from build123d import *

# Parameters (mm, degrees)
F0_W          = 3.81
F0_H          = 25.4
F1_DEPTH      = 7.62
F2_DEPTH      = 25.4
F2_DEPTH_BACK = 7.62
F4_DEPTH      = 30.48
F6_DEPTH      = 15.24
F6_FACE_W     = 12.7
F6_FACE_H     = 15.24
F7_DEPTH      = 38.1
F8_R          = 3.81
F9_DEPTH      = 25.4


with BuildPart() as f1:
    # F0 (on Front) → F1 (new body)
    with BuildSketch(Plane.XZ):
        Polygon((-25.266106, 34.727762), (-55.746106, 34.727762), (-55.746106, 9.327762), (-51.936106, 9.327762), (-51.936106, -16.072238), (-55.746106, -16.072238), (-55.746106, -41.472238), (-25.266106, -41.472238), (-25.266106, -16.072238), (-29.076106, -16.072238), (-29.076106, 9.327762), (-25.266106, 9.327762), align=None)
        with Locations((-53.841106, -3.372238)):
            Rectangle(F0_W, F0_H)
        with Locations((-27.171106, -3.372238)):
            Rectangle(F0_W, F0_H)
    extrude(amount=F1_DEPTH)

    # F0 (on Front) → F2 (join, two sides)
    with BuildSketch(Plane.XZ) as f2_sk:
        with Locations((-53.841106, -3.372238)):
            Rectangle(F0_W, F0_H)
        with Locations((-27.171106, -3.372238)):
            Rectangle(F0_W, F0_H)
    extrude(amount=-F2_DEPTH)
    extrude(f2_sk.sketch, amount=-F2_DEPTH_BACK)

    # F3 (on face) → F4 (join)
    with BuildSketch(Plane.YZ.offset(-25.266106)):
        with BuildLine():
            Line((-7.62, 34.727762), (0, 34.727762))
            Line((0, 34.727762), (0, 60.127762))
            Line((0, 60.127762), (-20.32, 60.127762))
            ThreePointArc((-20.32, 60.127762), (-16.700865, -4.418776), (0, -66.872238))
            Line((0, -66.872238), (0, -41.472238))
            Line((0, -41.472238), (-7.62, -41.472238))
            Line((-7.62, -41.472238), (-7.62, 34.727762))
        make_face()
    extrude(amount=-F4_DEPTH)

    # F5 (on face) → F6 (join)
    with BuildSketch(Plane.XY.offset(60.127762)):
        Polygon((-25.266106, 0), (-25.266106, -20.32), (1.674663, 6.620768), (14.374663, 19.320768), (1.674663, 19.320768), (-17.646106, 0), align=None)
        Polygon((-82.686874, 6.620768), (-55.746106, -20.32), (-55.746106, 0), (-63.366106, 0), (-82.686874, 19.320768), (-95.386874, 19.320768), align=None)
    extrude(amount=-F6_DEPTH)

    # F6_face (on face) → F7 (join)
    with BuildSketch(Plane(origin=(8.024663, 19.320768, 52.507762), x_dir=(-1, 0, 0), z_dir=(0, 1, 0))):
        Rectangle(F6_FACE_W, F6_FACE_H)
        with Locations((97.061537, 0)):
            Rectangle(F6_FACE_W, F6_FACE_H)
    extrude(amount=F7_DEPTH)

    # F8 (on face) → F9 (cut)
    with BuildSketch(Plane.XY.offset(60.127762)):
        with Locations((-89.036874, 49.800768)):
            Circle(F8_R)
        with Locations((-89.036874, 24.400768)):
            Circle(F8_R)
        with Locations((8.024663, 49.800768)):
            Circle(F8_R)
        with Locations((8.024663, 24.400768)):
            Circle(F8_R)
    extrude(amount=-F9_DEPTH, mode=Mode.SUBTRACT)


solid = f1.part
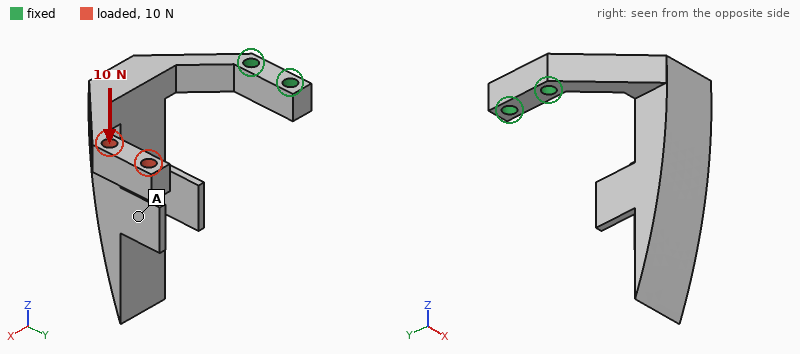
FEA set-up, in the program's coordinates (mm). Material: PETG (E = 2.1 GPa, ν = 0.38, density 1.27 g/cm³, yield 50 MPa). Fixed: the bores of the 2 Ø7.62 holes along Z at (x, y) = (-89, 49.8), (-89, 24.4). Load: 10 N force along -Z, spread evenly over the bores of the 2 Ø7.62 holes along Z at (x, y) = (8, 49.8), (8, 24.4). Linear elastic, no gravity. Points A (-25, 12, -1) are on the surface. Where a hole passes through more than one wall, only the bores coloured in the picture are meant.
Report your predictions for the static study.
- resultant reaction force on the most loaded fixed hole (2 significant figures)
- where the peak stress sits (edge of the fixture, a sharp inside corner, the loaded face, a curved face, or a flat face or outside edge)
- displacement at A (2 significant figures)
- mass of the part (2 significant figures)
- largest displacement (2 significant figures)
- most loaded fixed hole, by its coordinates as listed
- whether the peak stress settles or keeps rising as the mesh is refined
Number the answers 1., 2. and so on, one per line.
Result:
1. 9.7 N
2. edge of the fixture
3. 1.2 mm
4. 110 g
5. 2.1 mm
6. (-89, 24.4)
7. keeps rising
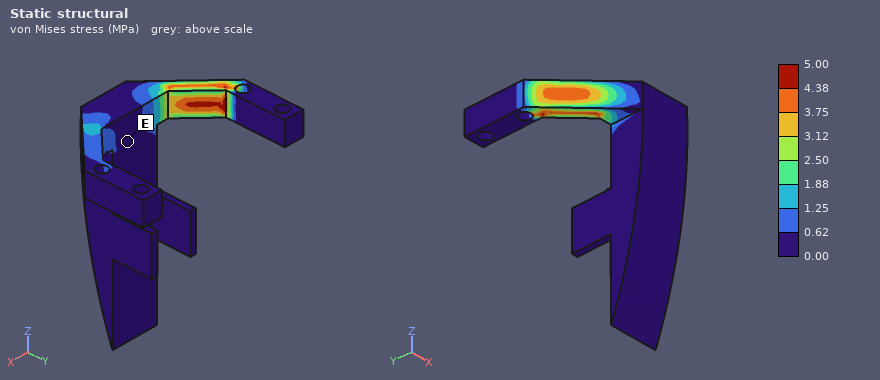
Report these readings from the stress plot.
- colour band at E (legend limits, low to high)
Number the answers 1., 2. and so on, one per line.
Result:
1. 0.00 to 0.62 MPa
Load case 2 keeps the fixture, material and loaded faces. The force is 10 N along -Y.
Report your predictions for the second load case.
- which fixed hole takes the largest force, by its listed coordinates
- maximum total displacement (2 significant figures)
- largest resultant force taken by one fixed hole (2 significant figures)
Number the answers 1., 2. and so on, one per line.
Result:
1. (-89, 24.4)
2. 1.9 mm
3. 9.6 N
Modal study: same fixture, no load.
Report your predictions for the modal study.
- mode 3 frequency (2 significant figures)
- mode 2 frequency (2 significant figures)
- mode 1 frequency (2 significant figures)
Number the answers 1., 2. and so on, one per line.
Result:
1. 120 Hz
2. 79 Hz
3. 56 Hz
